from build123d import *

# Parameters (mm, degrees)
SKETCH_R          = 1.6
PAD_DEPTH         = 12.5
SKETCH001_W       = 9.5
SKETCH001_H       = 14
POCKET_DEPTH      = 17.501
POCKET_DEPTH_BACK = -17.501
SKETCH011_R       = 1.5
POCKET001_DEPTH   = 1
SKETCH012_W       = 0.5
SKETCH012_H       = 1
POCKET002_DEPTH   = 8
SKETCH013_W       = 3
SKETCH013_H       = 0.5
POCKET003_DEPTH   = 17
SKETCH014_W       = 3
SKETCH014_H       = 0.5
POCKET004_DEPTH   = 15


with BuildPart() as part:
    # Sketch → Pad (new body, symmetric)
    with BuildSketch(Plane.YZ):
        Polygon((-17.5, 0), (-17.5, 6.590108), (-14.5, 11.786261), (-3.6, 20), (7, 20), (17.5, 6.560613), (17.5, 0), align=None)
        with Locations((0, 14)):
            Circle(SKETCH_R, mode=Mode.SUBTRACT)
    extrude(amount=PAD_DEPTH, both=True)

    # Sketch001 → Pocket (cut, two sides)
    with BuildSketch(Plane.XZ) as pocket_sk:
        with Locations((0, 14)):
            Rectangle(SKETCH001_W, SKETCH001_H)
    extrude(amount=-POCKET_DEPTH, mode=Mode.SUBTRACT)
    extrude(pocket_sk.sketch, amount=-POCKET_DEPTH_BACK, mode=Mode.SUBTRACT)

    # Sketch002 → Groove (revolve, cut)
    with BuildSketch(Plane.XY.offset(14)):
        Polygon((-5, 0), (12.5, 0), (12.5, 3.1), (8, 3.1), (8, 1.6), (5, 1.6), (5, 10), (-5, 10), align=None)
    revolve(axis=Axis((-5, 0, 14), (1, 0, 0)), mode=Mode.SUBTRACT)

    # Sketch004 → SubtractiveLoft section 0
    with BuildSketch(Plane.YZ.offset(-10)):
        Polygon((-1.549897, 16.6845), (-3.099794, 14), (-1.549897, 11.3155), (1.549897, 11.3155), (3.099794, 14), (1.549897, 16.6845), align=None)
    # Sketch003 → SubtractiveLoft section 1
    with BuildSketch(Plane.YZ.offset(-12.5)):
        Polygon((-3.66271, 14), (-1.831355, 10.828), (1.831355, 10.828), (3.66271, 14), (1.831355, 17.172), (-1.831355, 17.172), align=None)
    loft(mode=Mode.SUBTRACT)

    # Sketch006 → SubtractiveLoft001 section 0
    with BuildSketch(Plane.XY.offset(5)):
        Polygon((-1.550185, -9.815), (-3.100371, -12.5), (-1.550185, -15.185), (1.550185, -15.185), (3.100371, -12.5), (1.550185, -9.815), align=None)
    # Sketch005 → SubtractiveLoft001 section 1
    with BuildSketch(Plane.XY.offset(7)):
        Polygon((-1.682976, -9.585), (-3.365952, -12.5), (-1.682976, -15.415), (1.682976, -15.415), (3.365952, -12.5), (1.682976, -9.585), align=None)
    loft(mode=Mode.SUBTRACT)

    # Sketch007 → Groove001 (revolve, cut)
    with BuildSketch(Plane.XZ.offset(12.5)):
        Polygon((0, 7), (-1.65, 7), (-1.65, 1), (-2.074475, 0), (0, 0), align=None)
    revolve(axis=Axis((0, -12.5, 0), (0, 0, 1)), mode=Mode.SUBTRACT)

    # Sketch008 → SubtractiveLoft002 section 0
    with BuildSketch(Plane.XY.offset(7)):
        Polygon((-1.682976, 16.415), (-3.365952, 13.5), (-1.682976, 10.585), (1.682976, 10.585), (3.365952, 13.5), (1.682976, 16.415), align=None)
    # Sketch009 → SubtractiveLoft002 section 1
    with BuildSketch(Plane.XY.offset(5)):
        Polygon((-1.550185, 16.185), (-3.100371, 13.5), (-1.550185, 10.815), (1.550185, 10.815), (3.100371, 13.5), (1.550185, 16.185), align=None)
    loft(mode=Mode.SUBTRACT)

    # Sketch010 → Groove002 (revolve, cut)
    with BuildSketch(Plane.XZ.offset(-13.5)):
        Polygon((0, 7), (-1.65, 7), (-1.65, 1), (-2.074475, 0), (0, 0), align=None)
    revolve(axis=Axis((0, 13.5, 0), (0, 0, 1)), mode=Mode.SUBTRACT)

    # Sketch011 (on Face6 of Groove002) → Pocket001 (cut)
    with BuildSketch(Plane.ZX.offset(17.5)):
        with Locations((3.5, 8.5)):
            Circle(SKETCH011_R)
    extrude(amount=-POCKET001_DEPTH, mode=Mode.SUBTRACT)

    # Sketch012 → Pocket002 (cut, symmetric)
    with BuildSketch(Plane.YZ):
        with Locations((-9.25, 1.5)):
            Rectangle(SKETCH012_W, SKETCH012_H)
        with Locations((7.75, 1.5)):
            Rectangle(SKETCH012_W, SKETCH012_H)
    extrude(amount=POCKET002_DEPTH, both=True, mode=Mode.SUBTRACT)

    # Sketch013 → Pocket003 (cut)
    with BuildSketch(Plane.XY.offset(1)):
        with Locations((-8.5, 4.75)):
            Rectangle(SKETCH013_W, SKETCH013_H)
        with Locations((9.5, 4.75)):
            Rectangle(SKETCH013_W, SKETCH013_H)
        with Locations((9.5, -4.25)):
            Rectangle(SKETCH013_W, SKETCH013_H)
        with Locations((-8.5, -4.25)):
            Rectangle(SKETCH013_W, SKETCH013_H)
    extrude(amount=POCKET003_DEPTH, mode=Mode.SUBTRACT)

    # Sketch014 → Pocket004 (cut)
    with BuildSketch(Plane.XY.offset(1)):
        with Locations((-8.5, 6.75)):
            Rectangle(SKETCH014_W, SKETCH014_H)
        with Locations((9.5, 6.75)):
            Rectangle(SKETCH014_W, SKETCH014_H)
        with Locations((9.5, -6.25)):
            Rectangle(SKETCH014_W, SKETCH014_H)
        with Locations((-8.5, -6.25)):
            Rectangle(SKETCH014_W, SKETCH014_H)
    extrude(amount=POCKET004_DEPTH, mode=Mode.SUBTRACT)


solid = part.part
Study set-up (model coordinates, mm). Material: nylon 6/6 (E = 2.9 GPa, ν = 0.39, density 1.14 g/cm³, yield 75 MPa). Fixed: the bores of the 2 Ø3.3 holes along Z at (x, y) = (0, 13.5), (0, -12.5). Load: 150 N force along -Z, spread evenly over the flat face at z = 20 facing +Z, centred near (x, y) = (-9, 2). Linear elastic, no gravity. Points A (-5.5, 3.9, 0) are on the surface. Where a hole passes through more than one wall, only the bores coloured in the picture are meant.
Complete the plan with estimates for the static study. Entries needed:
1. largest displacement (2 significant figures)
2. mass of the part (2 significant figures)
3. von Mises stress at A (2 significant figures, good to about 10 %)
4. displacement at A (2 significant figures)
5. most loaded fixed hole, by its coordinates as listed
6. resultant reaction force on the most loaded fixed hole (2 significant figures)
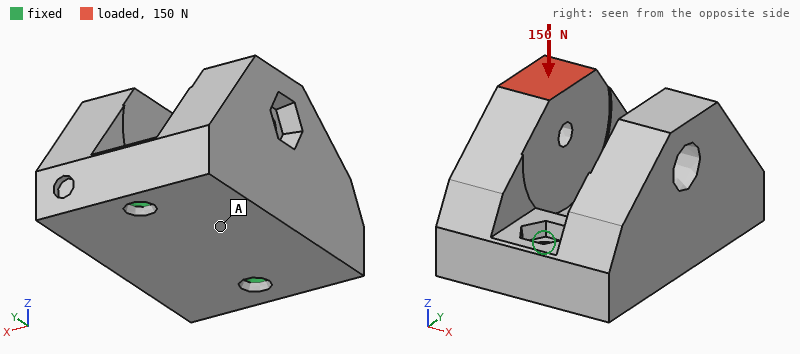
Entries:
0.14 mm
11 g
1.7 MPa
0.039 mm
(0, 13.5)
83 N
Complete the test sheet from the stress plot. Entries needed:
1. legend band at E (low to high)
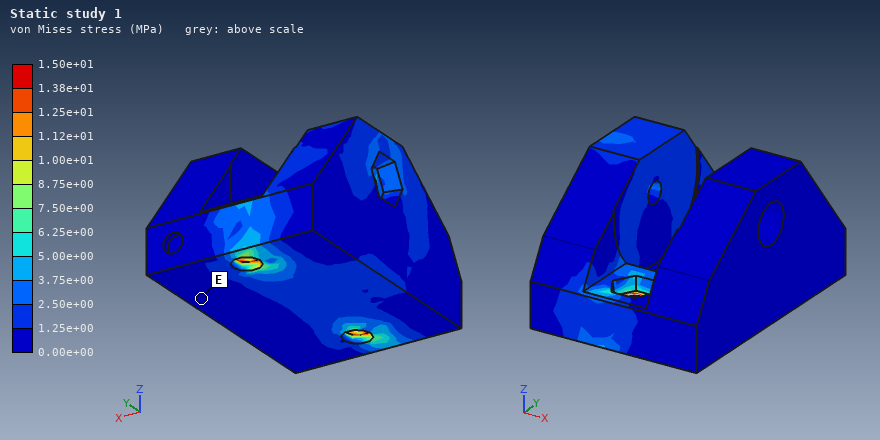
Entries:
0.00e+00 to 1.25e+00 MPa
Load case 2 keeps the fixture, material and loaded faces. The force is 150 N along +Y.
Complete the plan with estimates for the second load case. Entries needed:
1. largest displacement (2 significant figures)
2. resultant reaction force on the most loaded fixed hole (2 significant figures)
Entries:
64 µm
130 N
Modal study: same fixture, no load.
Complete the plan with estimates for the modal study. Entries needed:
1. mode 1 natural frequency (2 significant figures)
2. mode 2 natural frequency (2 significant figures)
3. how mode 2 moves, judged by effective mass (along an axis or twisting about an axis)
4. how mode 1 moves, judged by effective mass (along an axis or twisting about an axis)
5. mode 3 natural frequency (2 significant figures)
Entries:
2300 Hz
3800 Hz
along Z
along X
6100 Hz
